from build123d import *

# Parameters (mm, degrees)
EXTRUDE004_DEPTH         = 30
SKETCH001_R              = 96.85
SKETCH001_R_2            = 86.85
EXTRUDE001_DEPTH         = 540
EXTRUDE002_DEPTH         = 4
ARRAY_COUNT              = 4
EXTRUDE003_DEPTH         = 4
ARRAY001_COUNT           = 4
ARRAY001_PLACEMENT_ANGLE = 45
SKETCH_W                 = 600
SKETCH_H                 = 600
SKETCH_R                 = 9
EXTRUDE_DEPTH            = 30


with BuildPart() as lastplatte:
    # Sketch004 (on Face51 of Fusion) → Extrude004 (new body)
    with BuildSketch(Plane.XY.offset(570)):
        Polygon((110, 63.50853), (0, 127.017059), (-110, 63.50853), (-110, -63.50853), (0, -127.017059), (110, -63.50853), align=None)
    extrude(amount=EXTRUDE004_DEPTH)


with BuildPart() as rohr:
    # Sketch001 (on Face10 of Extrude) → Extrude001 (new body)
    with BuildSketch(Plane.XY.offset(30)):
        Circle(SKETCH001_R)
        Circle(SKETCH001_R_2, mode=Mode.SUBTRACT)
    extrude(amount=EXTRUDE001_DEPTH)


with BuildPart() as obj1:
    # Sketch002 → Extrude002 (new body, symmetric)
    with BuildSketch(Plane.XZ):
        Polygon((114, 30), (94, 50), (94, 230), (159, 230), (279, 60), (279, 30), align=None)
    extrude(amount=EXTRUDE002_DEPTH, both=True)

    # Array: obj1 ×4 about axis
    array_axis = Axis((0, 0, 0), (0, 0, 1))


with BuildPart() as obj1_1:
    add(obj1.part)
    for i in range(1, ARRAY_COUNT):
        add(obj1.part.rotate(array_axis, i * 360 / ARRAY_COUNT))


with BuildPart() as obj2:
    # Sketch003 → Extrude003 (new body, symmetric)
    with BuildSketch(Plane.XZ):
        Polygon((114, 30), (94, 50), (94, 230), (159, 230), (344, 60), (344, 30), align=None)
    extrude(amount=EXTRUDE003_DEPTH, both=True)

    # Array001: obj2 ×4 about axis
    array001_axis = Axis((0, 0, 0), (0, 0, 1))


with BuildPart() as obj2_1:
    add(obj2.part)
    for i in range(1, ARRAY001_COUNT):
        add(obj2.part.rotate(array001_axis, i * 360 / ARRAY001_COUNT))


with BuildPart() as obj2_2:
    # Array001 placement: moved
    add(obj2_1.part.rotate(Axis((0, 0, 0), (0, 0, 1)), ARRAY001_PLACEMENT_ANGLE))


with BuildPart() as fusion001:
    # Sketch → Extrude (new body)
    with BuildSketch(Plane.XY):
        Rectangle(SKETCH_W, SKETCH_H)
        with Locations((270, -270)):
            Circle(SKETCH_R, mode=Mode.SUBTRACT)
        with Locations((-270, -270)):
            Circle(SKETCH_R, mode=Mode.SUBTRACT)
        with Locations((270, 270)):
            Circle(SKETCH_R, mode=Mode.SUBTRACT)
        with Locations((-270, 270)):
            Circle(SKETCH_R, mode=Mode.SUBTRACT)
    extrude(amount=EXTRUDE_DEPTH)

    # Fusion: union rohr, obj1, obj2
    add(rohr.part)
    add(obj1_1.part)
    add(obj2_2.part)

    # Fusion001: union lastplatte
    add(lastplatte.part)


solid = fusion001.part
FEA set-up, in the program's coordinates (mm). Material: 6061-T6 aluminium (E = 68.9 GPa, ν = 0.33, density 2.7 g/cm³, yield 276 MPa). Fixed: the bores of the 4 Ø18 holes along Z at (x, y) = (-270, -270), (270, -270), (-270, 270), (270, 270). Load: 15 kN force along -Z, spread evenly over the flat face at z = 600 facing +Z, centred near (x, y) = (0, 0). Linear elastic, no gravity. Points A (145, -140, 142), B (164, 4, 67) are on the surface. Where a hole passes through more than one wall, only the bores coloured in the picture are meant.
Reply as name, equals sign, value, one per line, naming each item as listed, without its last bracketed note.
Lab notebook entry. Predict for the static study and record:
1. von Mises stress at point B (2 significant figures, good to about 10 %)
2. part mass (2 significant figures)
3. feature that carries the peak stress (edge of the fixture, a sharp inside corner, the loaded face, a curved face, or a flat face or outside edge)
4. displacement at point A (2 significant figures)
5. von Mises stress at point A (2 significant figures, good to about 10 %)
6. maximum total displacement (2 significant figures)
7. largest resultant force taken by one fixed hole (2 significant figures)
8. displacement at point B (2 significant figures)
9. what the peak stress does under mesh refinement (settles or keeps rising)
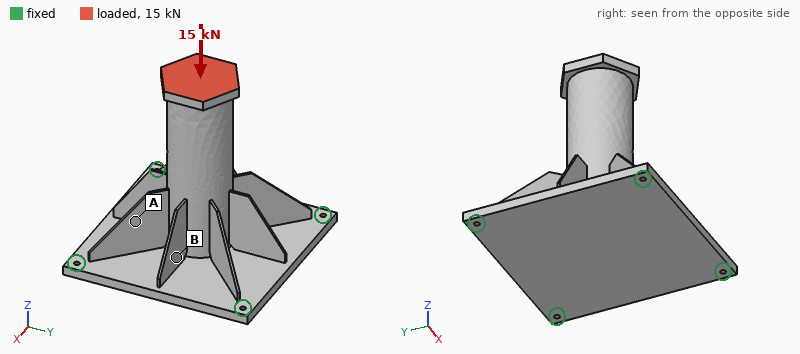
von Mises stress at point B = 2.0 MPa
part mass = 46 kg
feature that carries the peak stress = edge of the fixture
displacement at point A = 53 µm
von Mises stress at point A = 5.1 MPa
maximum total displacement = 87 µm
largest resultant force taken by one fixed hole = 4.2 kN
displacement at point B = 65 µm
what the peak stress does under mesh refinement = keeps rising
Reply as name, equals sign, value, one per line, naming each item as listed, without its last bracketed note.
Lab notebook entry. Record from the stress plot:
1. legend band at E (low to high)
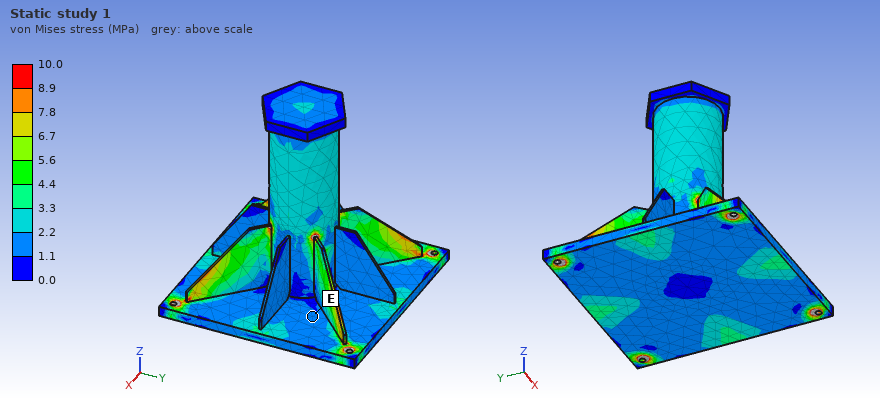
legend band at E = 1.1 to 2.2 MPa
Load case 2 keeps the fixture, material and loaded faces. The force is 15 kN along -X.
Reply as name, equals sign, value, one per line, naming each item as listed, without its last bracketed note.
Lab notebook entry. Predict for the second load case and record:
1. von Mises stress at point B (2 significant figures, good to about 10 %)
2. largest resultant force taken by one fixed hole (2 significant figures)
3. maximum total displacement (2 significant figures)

von Mises stress at point B = 6.4 MPa
largest resultant force taken by one fixed hole = 10.0 kN
maximum total displacement = 0.77 mm
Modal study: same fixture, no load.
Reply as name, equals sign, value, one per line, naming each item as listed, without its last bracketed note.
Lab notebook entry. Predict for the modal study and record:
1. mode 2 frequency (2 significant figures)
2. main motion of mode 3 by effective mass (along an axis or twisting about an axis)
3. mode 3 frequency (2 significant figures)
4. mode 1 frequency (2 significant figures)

mode 2 frequency = 300 Hz
main motion of mode 3 by effective mass = along Z
mode 3 frequency = 400 Hz
mode 1 frequency = 300 Hz
